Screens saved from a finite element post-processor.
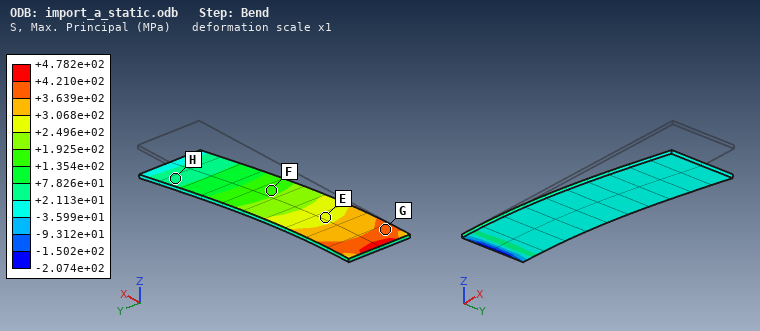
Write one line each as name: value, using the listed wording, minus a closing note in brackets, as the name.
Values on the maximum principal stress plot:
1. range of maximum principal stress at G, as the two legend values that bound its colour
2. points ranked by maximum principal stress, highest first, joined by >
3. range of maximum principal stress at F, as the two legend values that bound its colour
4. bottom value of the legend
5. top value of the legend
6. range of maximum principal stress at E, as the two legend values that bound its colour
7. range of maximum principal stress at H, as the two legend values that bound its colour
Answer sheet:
range of maximum principal stress at G, as the two legend values that bound its colour: +3.639e+02 to +4.210e+02 MPa
points ranked by maximum principal stress, highest first, joined by >: G > E > F > H
range of maximum principal stress at F, as the two legend values that bound its colour: +1.354e+02 to +1.925e+02 MPa
bottom value of the legend: -2.074e+02 MPa
top value of the legend: +4.782e+02 MPa
range of maximum principal stress at E, as the two legend values that bound its colour: +2.496e+02 to +3.068e+02 MPa
range of maximum principal stress at H, as the two legend values that bound its colour: +2.113e+01 to +7.826e+01 MPa
